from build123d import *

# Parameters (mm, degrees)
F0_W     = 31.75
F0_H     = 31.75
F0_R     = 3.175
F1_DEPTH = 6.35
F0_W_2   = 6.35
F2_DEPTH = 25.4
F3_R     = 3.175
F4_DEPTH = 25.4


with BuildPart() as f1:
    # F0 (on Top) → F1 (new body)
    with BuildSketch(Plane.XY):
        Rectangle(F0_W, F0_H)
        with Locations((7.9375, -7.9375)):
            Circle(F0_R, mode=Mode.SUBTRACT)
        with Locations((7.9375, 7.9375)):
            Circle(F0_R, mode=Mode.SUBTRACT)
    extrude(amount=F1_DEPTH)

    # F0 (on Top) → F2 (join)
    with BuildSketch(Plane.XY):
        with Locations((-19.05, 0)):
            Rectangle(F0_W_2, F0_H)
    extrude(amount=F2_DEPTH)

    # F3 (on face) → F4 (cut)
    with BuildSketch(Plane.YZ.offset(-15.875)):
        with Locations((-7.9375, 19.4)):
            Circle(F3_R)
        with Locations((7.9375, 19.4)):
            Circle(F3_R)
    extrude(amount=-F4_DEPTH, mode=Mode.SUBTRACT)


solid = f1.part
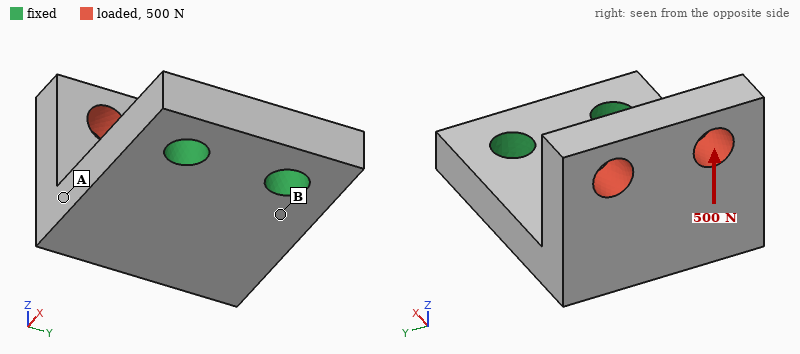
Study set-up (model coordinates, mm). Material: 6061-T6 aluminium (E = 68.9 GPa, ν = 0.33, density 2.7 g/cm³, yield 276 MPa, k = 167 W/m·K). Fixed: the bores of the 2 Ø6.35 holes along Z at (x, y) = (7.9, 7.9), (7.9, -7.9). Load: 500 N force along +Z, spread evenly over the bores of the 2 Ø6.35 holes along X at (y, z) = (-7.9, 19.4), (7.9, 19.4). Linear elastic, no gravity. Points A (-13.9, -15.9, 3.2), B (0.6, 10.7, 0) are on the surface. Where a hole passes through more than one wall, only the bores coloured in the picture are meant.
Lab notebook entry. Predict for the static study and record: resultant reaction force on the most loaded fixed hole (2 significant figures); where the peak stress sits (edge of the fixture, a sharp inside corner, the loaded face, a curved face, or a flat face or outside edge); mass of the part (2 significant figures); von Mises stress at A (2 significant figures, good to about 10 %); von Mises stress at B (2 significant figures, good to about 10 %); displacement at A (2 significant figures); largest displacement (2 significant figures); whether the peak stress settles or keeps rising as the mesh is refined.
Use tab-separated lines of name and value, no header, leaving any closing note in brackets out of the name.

resultant reaction force on the most loaded fixed hole	250 N
where the peak stress sits	edge of the fixture
mass of the part	29 g
von Mises stress at A	13 MPa
von Mises stress at B	44 MPa
displacement at A	0.040 mm
largest displacement	0.10 mm
whether the peak stress settles or keeps rising as the mesh is refined	keeps rising
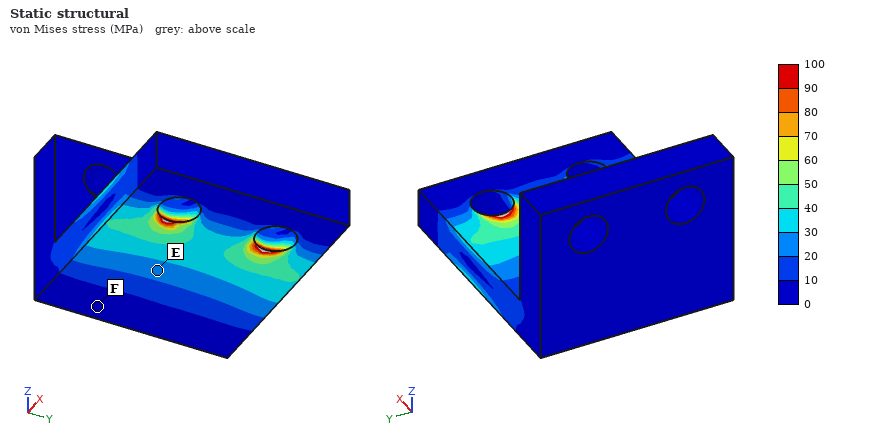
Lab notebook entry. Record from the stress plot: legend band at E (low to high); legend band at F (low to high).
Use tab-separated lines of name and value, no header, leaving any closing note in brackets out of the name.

legend band at E	20 to 30 MPa
legend band at F	0 to 10 MPa
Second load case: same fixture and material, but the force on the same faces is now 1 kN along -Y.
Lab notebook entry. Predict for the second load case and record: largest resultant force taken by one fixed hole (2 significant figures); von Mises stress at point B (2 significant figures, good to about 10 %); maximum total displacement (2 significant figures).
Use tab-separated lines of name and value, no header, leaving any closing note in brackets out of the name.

largest resultant force taken by one fixed hole	1.5 kN
von Mises stress at point B	56 MPa
maximum total displacement	0.12 mm
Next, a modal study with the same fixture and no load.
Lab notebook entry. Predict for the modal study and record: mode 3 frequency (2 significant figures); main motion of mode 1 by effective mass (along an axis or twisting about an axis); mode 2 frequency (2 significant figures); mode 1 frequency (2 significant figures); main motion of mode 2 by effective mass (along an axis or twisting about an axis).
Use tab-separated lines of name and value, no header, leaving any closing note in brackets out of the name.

mode 3 frequency	9400 Hz
main motion of mode 1 by effective mass	along Z
mode 2 frequency	5600 Hz
mode 1 frequency	3200 Hz
main motion of mode 2 by effective mass	along Y
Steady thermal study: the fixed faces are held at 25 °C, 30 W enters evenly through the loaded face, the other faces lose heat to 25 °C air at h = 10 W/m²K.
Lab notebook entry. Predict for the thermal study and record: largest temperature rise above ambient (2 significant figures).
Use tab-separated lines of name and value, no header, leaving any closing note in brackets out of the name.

largest temperature rise above ambient	38 K
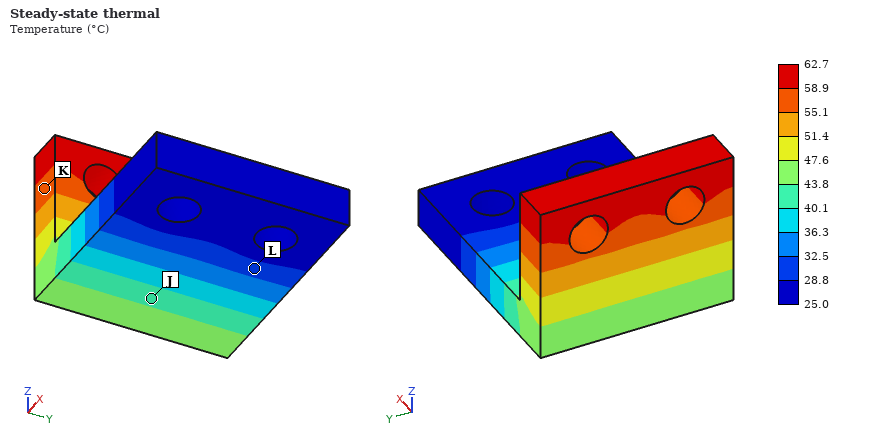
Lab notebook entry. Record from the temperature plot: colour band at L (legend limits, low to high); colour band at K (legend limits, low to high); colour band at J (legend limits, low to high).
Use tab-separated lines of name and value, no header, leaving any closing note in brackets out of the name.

colour band at L	28.8 to 32.5 °C
colour band at K	55.1 to 58.9 °C
colour band at J	40.1 to 43.8 °C
